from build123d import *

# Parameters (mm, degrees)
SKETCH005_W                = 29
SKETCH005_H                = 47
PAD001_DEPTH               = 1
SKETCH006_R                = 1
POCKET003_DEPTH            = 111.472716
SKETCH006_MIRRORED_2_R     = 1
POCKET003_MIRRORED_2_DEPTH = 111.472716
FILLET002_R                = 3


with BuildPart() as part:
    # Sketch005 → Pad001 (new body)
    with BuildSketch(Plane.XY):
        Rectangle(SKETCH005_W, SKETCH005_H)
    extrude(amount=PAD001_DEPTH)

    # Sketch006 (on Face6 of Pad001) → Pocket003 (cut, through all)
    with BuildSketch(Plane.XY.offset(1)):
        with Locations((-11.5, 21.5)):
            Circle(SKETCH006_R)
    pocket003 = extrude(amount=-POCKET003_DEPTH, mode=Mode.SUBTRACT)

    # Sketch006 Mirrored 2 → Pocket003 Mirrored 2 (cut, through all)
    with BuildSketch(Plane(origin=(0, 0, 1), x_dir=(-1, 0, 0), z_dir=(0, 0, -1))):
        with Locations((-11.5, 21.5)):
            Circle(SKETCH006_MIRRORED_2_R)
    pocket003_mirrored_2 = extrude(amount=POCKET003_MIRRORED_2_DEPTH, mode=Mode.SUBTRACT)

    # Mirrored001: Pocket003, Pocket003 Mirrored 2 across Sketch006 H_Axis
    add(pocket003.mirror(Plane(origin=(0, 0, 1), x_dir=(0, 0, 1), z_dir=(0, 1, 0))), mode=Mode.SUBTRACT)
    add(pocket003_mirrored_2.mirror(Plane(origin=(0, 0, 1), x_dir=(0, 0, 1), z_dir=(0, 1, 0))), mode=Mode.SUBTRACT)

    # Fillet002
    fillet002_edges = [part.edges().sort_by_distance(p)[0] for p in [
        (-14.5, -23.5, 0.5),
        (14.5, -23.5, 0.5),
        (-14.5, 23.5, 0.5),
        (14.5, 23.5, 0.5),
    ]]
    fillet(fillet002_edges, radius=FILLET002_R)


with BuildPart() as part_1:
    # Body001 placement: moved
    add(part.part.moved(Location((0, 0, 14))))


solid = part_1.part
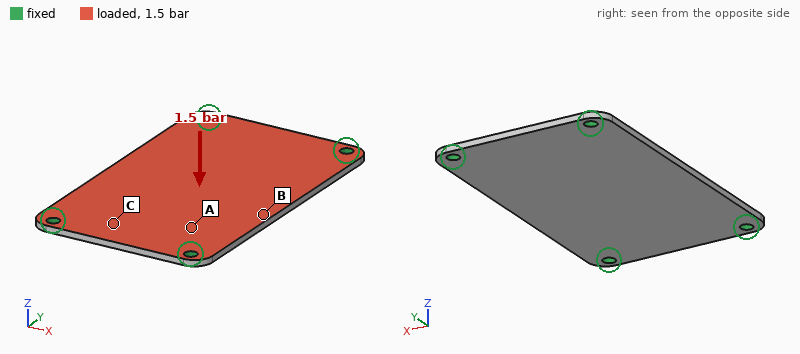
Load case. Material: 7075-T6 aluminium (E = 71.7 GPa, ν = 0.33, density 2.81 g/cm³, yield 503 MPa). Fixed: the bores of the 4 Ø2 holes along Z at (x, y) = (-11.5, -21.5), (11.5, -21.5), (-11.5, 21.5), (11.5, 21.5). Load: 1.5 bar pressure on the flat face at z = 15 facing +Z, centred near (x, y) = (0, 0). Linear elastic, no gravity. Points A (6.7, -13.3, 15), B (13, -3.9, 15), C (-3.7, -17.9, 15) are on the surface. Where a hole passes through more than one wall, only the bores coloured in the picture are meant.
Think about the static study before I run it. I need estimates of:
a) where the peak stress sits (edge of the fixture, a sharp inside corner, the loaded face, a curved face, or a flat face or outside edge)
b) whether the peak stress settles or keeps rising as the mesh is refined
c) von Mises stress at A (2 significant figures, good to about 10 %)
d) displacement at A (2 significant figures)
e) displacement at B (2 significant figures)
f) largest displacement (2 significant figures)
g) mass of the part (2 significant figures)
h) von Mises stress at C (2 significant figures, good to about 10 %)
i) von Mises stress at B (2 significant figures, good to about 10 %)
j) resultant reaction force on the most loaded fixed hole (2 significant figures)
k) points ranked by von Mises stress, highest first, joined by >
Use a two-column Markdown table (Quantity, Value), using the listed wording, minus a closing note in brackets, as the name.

| Quantity | Value |
|---|---|
| where the peak stress sits | edge of the fixture |
| whether the peak stress settles or keeps rising as the mesh is refined | keeps rising |
| von Mises stress at A | 19 MPa |
| displacement at A | 0.12 mm |
| displacement at B | 0.25 mm |
| largest displacement | 0.27 mm |
| mass of the part | 3.8 g |
| von Mises stress at C | 38 MPa |
| von Mises stress at B | 76 MPa |
| resultant reaction force on the most loaded fixed hole | 50 N |
| points ranked by von Mises stress, highest first, joined by > | B > C > A |
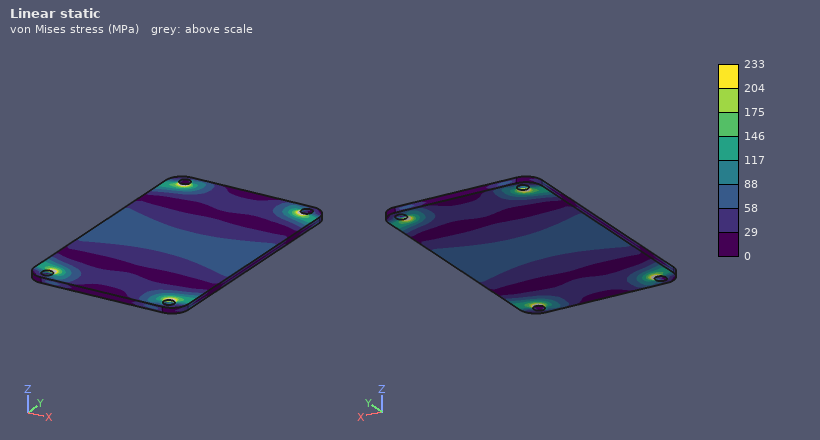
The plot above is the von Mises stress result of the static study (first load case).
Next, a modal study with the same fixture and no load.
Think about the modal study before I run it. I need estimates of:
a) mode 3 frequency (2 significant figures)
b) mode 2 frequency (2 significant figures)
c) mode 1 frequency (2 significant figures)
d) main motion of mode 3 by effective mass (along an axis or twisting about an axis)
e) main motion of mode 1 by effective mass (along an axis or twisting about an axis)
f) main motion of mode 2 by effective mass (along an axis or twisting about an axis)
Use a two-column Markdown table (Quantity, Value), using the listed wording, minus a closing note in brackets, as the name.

| Quantity | Value |
|---|---|
| mode 3 frequency | 6900 Hz |
| mode 2 frequency | 4000 Hz |
| mode 1 frequency | 2600 Hz |
| main motion of mode 3 by effective mass | twisting about X |
| main motion of mode 1 by effective mass | along Z |
| main motion of mode 2 by effective mass | twisting about Y |
